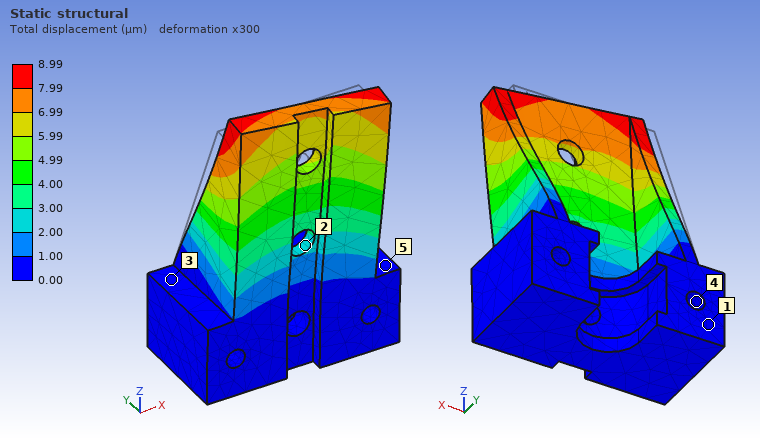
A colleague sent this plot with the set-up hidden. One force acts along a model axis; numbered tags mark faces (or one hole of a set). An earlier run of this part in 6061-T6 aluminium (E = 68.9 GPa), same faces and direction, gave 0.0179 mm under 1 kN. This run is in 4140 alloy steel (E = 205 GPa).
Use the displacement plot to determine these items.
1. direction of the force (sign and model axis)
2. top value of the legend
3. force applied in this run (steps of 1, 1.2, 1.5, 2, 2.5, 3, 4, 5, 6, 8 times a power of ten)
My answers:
+X
8.99 µm
1.5 kN
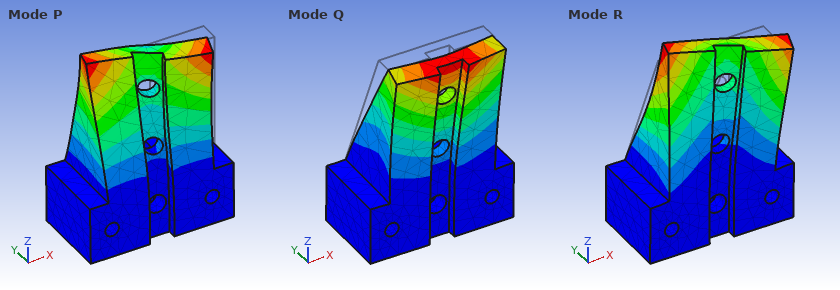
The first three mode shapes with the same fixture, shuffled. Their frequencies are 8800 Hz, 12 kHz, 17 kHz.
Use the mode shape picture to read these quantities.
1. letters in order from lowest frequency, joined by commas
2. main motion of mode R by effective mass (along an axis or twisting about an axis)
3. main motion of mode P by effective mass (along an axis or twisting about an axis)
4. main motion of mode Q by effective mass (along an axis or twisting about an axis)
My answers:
Q, R, P
along X
along X
along Y
